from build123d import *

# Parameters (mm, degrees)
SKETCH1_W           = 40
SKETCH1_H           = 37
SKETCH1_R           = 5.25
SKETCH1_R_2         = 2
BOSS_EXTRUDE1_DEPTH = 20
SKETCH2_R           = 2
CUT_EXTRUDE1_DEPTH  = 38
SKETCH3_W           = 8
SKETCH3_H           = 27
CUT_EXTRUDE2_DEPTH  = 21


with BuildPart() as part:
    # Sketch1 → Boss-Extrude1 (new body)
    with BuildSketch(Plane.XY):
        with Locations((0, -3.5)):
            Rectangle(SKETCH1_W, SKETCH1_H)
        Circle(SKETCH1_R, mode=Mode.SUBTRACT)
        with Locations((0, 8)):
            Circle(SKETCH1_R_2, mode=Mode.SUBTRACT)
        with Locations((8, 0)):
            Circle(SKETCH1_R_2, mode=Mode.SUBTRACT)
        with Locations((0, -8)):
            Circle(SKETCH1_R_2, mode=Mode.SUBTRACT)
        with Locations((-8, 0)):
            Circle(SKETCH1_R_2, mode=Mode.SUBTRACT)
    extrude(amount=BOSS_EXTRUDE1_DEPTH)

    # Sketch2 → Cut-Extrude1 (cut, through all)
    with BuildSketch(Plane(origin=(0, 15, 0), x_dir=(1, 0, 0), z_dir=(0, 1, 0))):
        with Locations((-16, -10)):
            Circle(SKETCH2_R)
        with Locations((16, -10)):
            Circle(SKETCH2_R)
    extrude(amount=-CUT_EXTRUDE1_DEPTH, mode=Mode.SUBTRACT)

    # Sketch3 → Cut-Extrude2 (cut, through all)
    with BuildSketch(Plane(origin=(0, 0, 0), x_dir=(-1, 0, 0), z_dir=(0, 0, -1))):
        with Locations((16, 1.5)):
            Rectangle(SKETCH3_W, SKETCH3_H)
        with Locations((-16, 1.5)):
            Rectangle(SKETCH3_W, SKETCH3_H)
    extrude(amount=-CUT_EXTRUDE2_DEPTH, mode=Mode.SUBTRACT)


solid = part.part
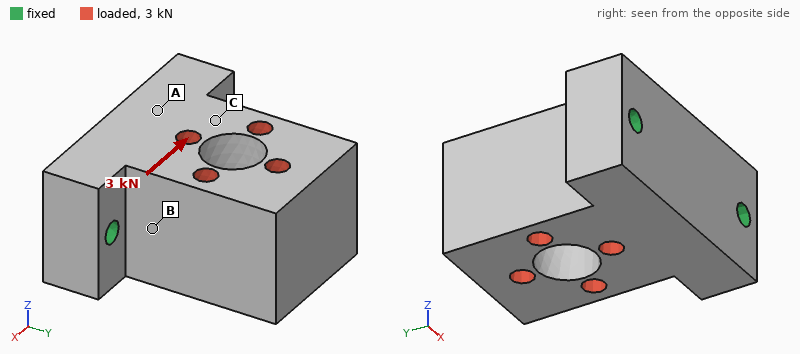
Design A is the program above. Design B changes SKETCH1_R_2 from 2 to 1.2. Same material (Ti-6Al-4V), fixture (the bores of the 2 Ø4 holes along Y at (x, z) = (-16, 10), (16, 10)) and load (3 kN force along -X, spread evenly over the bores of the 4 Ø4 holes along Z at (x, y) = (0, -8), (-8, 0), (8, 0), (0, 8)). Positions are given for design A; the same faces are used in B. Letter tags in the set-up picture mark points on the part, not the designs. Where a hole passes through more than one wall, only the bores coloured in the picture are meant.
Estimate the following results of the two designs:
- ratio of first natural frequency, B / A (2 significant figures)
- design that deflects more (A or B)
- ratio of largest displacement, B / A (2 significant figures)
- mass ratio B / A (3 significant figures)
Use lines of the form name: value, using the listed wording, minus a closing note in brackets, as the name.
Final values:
ratio of first natural frequency, B / A: 0.99
design that deflects more: A
ratio of largest displacement, B / A: 0.79
mass ratio B / A: 1.04
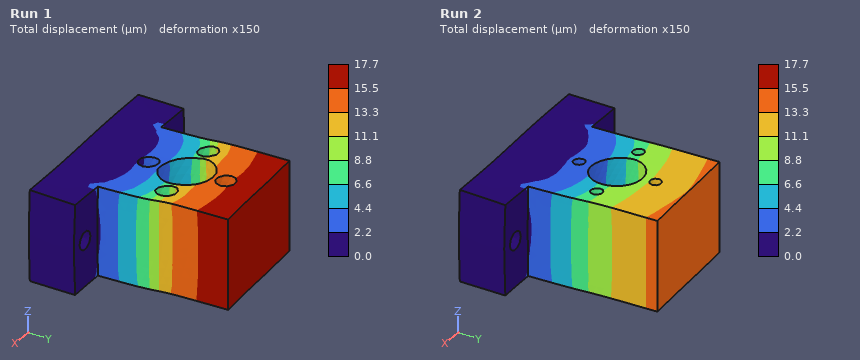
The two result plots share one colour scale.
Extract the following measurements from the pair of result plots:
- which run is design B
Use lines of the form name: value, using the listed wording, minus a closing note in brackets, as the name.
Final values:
which run is design B: Run 2
